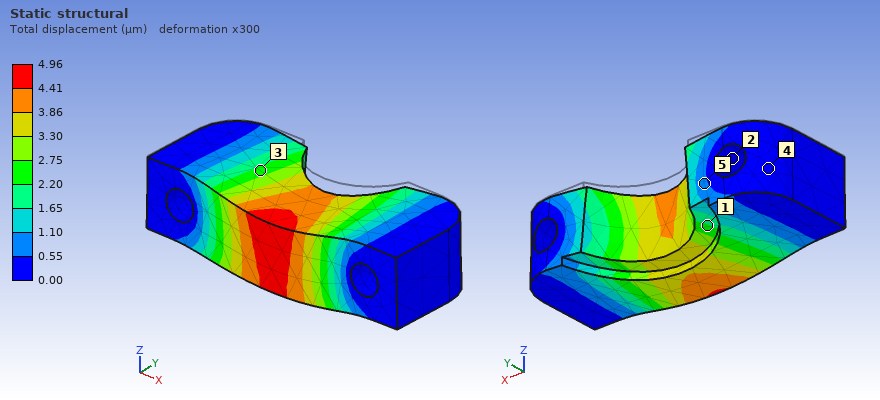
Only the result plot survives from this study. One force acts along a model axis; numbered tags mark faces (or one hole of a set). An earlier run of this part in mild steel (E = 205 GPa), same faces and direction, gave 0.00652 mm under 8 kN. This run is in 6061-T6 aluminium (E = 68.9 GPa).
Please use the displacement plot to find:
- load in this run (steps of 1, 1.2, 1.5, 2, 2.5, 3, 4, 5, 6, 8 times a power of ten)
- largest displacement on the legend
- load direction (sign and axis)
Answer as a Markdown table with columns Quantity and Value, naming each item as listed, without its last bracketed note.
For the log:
| Quantity | Value |
|---|---|
| load in this run | 2 kN |
| largest displacement on the legend | 4.96 µm |
| load direction | -Z |
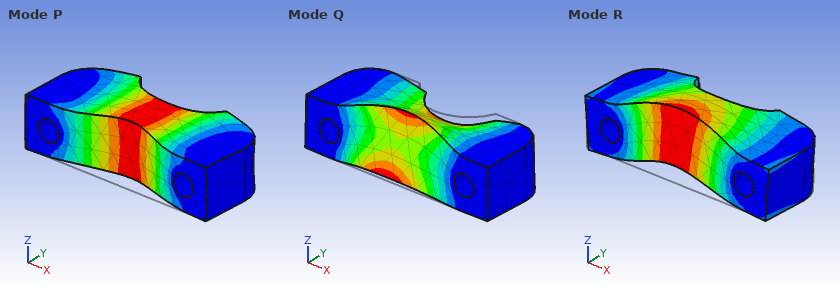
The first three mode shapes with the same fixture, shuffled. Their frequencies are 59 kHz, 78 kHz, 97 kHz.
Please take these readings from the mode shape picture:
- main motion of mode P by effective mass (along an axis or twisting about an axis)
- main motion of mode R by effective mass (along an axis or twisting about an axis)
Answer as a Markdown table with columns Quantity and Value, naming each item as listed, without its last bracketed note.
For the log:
| Quantity | Value |
|---|---|
| main motion of mode P by effective mass | along Y |
| main motion of mode R by effective mass | along Z |
